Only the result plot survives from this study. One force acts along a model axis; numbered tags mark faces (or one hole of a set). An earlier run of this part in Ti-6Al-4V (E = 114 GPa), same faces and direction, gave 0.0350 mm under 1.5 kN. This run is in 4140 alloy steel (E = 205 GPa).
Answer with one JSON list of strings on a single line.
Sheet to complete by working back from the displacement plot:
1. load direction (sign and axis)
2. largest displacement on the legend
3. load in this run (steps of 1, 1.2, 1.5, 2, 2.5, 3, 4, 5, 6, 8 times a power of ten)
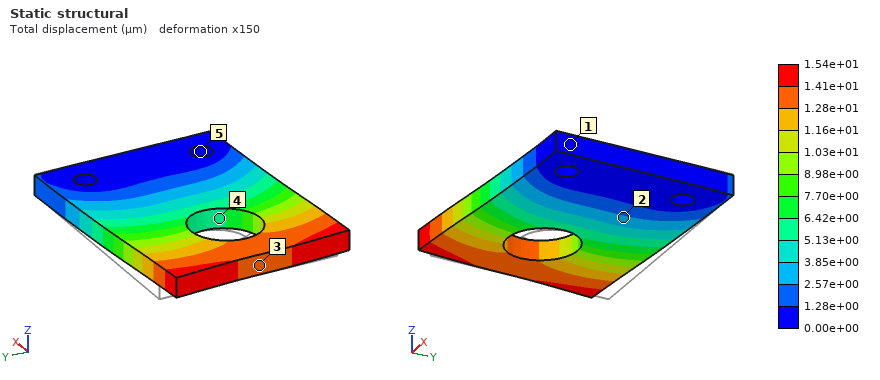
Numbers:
["-Y", "1.54e+01 µm", "1.2 kN"]
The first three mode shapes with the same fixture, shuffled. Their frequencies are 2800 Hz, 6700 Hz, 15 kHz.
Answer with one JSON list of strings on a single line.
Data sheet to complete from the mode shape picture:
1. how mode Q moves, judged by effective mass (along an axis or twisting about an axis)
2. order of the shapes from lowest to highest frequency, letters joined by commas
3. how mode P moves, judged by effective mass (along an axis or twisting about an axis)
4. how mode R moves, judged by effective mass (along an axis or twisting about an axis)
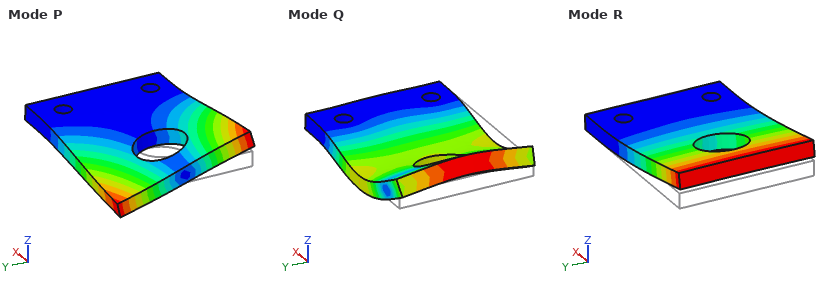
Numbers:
["along Z", "R, P, Q", "twisting about X", "along Z"]
